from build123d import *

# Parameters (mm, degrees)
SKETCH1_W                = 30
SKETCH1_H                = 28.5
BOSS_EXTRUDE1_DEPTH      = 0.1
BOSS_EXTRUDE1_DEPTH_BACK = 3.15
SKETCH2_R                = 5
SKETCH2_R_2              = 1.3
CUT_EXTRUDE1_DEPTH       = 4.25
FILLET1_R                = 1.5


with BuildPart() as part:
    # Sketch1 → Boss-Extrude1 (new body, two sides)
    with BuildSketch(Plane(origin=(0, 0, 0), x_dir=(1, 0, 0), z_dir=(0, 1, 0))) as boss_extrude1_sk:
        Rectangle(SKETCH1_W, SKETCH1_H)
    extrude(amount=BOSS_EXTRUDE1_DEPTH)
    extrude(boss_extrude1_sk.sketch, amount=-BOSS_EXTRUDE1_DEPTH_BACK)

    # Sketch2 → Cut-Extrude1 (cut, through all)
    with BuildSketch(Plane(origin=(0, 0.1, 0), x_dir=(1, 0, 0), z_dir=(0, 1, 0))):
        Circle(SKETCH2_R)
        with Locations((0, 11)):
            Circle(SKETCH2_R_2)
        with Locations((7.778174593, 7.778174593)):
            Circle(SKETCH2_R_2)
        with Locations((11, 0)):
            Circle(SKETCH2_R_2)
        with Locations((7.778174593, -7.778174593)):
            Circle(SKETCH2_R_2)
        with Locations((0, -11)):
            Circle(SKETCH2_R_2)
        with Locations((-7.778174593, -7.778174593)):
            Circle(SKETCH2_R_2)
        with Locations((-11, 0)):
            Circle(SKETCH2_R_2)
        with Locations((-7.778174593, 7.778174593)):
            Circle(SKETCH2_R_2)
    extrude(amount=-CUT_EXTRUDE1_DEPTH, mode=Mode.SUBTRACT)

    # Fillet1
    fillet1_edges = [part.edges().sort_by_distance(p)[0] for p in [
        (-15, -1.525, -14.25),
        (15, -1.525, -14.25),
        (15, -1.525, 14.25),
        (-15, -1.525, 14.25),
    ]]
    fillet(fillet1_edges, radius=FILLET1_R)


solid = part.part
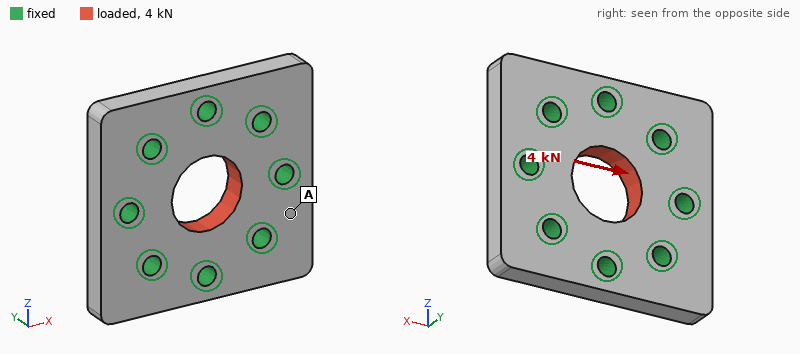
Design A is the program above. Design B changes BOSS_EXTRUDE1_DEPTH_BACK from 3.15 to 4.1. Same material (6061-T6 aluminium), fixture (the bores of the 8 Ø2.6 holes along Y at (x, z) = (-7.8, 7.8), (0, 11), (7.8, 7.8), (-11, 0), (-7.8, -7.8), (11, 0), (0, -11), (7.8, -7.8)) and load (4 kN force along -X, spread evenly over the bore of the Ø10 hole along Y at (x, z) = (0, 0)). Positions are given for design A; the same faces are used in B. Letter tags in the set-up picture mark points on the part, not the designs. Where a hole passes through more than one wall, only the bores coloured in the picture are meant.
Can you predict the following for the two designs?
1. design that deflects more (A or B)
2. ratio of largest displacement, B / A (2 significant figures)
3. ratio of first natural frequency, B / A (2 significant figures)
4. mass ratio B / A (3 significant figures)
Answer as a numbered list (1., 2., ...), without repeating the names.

1. A
2. 0.78
3. 1.2
4. 1.29
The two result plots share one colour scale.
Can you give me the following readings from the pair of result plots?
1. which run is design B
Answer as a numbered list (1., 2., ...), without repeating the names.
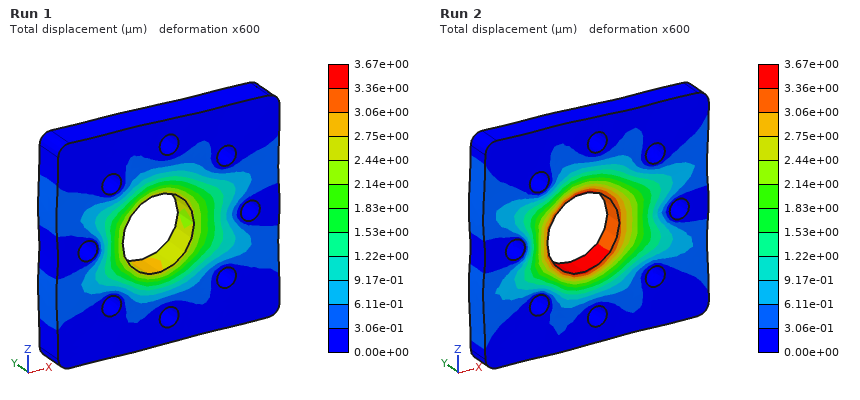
1. Run 1
